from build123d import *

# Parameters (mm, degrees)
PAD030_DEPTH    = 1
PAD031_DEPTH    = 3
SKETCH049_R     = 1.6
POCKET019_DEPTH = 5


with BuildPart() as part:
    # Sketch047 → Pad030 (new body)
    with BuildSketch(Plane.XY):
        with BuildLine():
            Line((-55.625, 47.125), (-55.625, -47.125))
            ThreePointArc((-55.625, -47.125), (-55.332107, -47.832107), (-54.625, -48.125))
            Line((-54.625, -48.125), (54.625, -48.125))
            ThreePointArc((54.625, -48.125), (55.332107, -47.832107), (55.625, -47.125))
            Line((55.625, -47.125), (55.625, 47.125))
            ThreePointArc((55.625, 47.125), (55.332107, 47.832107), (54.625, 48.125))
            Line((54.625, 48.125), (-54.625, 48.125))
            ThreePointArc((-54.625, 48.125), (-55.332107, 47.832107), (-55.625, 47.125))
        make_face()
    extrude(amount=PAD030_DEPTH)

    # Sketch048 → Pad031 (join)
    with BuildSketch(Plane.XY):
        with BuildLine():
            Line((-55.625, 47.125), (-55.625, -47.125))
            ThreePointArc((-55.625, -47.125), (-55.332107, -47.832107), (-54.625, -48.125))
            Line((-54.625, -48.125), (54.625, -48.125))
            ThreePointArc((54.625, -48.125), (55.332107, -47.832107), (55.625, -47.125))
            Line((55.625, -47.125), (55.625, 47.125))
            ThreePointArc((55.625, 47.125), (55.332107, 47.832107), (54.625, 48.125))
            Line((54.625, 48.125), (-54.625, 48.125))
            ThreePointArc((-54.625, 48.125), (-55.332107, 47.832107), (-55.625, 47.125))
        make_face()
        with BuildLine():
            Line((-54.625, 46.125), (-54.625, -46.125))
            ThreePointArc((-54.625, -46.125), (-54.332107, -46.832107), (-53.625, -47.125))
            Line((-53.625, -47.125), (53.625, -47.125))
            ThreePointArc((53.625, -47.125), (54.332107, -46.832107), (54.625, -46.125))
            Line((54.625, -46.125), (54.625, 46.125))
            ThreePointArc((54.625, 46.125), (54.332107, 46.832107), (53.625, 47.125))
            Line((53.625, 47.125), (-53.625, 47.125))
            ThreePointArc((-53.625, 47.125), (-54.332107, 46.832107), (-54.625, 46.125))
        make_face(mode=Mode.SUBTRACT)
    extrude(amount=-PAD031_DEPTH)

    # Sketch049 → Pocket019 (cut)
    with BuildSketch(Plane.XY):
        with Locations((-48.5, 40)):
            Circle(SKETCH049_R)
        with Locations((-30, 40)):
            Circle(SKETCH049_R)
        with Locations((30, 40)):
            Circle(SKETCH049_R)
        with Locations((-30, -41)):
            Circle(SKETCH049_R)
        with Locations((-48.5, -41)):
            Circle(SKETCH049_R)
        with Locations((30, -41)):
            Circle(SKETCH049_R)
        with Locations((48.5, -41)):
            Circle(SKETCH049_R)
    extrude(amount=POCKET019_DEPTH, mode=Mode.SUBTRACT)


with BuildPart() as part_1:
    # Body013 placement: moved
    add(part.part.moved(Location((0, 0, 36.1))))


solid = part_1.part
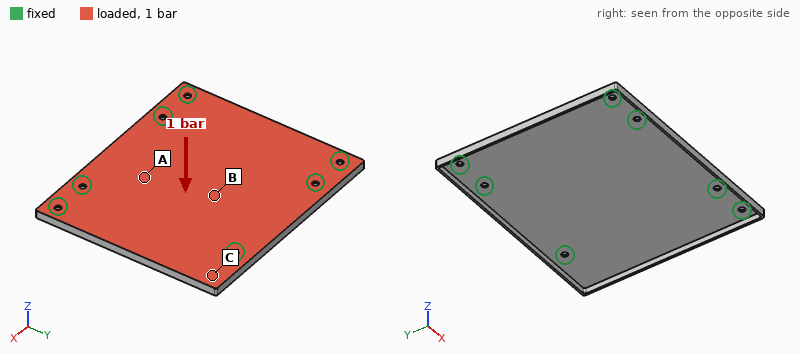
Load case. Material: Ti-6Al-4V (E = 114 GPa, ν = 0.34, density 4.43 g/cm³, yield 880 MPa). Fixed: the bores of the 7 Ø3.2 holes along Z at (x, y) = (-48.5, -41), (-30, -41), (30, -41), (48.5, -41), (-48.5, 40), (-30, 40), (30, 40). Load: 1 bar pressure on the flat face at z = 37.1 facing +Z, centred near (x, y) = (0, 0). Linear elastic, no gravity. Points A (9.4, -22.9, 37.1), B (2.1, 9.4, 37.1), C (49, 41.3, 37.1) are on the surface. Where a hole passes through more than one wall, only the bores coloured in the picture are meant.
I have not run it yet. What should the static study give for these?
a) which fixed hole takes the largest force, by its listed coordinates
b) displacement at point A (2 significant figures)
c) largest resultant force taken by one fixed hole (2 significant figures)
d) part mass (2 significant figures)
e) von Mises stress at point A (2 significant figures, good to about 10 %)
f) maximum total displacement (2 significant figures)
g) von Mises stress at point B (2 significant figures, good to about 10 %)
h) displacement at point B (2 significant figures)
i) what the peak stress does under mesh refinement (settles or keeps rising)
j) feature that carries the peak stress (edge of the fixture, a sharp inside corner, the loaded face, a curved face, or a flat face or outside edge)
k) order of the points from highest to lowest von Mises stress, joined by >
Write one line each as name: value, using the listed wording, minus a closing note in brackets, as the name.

which fixed hole takes the largest force, by its listed coordinates: (30, 40)
displacement at point A: 1.0 mm
largest resultant force taken by one fixed hole: 300 N
part mass: 53 g
von Mises stress at point A: 92 MPa
maximum total displacement: 1.6 mm
von Mises stress at point B: 150 MPa
displacement at point B: 1.5 mm
what the peak stress does under mesh refinement: keeps rising
feature that carries the peak stress: edge of the fixture
order of the points from highest to lowest von Mises stress, joined by >: B > A > C
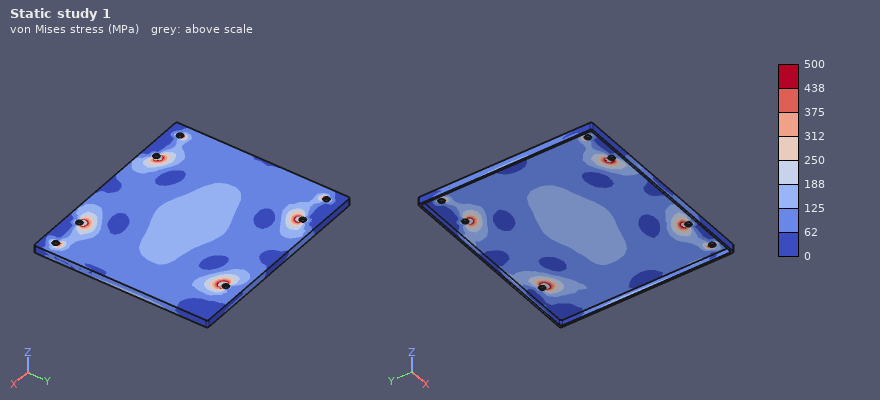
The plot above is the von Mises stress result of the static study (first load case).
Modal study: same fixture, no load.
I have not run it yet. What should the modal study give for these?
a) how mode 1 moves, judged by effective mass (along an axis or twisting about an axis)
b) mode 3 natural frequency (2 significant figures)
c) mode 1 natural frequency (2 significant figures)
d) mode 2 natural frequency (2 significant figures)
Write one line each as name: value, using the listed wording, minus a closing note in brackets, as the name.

how mode 1 moves, judged by effective mass: along Z
mode 3 natural frequency: 1400 Hz
mode 1 natural frequency: 750 Hz
mode 2 natural frequency: 1100 Hz
